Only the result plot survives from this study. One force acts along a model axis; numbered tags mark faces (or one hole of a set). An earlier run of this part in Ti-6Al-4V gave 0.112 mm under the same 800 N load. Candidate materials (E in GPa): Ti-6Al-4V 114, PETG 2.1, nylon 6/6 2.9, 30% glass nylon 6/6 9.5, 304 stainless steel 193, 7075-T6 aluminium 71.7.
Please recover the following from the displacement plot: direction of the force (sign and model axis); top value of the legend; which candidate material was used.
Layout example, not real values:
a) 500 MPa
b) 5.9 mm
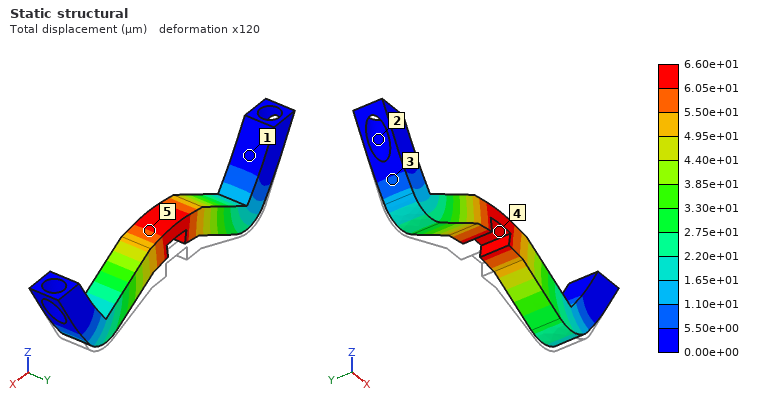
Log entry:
a) +Z
b) 6.60e+01 µm
c) 304 stainless steel
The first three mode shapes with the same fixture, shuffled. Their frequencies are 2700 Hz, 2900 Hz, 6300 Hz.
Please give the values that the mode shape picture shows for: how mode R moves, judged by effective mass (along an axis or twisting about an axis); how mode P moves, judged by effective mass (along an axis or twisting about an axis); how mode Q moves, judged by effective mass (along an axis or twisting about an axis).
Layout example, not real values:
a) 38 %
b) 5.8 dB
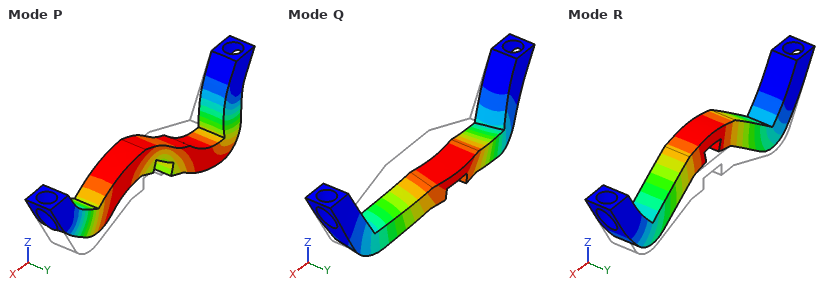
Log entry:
a) along Z
b) along X
c) along Y
